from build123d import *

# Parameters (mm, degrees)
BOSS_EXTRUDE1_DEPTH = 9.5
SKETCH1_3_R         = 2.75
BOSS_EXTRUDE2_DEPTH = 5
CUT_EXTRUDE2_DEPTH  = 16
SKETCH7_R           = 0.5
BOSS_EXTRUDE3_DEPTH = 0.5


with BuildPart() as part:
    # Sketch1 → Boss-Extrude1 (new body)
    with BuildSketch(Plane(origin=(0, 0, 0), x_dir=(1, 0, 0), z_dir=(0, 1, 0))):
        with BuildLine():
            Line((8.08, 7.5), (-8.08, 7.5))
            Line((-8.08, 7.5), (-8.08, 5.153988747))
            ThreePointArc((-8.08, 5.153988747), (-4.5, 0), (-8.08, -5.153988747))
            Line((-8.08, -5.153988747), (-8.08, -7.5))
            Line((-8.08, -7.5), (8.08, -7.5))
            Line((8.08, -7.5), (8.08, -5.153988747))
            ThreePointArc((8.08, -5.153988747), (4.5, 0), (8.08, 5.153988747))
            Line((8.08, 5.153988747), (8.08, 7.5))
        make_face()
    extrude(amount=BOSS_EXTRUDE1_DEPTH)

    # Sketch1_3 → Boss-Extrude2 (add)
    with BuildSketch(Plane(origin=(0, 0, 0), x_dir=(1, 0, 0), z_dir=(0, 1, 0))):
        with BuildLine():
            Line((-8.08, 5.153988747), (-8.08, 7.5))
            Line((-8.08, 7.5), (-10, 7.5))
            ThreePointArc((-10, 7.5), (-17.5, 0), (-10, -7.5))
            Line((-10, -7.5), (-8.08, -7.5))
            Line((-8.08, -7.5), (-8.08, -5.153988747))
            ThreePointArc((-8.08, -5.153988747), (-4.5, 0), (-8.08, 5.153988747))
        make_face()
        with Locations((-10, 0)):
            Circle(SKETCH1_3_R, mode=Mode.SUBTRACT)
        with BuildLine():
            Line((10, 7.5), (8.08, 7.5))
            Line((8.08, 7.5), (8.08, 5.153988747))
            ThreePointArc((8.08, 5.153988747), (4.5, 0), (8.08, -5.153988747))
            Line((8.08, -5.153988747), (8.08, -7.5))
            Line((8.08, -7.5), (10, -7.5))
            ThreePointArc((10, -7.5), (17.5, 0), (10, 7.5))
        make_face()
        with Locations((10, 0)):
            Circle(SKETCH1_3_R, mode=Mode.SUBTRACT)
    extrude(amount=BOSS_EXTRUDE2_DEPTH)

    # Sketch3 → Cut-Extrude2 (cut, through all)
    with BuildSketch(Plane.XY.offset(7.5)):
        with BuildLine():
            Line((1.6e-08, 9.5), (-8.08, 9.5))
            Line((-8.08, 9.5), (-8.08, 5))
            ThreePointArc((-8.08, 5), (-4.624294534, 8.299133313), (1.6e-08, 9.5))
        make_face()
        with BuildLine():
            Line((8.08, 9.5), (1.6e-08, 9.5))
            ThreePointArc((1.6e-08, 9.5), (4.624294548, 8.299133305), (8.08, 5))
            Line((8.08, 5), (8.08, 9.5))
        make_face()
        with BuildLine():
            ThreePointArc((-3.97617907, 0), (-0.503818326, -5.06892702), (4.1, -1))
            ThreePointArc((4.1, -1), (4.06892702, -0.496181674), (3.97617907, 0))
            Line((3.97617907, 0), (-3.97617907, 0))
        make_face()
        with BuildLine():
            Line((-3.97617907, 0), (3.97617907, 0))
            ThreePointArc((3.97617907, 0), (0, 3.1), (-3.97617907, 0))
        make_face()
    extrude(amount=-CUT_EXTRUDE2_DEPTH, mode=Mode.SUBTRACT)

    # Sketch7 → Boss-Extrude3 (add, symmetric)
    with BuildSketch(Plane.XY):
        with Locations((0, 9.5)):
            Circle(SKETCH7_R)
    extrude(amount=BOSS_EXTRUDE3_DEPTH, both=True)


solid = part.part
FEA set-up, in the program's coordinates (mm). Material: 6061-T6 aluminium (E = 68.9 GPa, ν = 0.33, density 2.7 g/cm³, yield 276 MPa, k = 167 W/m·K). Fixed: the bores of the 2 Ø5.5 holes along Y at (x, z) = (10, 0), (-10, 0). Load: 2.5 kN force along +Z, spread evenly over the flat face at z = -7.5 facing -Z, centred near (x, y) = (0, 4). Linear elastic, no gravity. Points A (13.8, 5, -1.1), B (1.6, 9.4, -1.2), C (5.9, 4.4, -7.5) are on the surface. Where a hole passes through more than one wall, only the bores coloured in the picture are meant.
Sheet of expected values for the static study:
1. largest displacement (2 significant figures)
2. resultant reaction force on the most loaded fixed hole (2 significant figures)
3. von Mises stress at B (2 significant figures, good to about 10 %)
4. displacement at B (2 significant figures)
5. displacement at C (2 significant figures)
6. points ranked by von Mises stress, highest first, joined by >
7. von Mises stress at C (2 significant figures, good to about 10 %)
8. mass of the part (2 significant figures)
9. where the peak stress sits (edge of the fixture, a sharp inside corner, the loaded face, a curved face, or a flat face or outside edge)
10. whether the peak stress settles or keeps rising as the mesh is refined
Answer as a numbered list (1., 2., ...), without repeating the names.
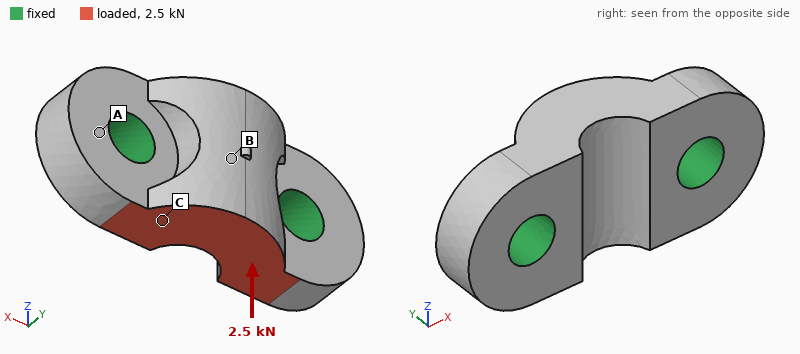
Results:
1. 13 µm
2. 1.3 kN
3. 18 MPa
4. 8.9 µm
5. 6.7 µm
6. C > B > A
7. 33 MPa
8. 6.9 g
9. edge of the fixture
10. keeps rising
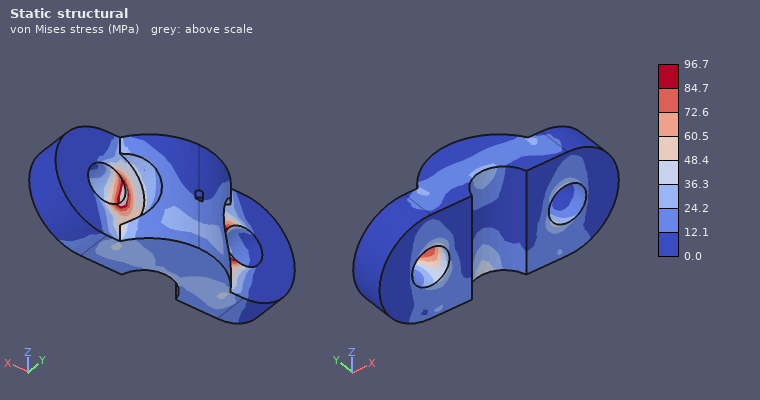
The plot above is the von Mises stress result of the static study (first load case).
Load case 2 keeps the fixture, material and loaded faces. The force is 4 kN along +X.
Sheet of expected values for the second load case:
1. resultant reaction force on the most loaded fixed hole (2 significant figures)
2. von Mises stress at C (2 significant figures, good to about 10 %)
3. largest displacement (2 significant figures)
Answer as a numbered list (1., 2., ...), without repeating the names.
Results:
1. 2.3 kN
2. 72 MPa
3. 13 µm
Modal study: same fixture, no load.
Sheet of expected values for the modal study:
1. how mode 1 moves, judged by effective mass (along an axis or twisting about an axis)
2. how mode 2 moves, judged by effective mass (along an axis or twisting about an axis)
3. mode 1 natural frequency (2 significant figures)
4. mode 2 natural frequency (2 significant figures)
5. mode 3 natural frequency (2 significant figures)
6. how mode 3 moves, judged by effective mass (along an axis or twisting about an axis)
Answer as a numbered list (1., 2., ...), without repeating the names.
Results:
1. along Z
2. along Y
3. 38 kHz
4. 55 kHz
5. 73 kHz
6. along Z
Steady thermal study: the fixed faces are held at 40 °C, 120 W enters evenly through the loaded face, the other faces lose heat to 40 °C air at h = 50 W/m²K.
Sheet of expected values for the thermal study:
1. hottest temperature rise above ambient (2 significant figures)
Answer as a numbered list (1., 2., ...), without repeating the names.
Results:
1. 52 K
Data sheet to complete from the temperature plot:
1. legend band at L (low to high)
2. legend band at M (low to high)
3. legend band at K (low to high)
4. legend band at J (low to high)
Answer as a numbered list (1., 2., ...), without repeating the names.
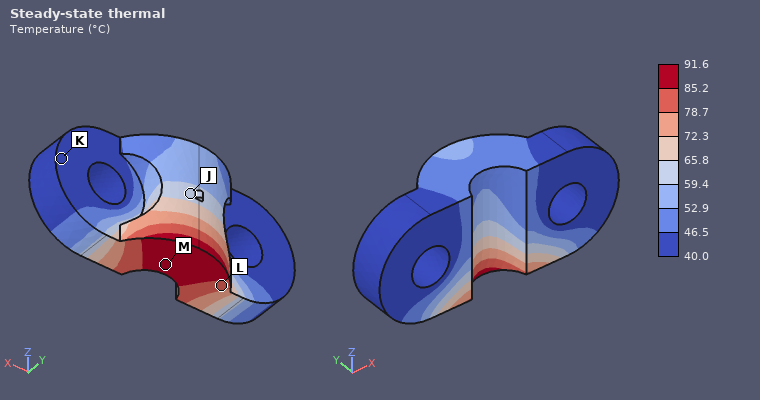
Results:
1. 78.7 to 85.2 °C
2. 85.2 to 91.6 °C
3. 40.0 to 46.5 °C
4. 59.4 to 65.8 °C
